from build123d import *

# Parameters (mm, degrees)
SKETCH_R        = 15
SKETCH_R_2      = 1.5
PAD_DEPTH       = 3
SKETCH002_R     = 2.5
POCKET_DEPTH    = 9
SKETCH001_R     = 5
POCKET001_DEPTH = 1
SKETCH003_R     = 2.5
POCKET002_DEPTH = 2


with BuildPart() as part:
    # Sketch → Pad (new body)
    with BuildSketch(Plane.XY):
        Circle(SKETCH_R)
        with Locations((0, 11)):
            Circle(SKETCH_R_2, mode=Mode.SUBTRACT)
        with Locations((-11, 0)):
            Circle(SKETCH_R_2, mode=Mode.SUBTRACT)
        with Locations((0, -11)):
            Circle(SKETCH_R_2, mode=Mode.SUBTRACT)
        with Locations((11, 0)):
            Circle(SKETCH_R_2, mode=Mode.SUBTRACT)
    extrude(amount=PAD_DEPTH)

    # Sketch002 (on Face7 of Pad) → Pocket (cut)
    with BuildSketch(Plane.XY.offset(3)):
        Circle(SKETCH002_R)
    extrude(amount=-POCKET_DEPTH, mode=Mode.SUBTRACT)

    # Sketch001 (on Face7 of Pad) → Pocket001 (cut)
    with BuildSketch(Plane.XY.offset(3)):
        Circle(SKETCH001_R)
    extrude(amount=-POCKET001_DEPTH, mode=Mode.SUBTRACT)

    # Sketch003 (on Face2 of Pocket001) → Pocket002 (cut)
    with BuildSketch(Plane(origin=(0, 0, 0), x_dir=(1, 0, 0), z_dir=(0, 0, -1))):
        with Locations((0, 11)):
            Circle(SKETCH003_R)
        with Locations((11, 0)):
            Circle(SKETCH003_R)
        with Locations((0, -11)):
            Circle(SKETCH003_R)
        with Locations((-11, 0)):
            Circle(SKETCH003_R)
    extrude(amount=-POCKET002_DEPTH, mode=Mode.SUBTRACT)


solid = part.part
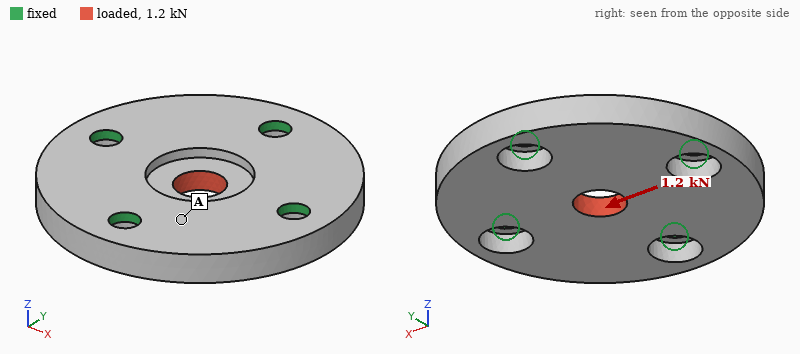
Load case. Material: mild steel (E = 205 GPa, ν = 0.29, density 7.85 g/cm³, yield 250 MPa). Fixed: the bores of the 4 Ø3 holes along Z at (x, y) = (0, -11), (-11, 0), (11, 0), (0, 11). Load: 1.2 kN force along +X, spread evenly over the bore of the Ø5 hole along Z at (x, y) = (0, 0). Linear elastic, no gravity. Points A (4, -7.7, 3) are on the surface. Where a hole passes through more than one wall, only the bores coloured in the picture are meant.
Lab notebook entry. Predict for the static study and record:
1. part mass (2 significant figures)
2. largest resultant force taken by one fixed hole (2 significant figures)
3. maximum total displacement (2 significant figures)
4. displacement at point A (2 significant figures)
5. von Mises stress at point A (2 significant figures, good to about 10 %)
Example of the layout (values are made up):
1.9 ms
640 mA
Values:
14 g
370 N
1.8 µm
0.51 µm
13 MPa
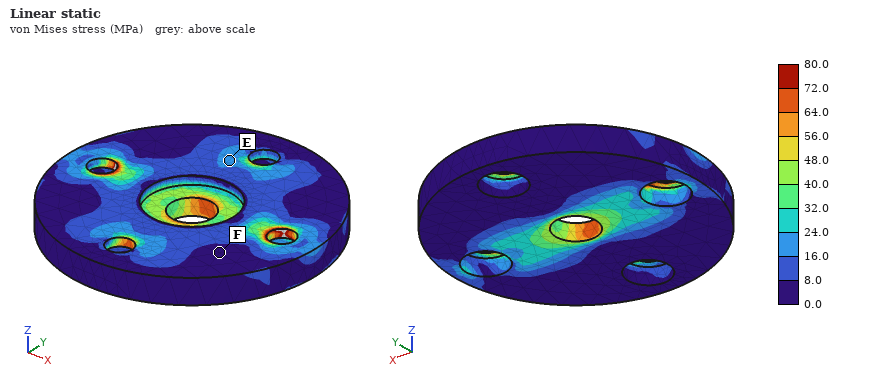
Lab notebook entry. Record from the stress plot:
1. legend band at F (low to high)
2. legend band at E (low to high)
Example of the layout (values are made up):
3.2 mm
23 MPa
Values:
0.0 to 8.0 MPa
16.0 to 24.0 MPa
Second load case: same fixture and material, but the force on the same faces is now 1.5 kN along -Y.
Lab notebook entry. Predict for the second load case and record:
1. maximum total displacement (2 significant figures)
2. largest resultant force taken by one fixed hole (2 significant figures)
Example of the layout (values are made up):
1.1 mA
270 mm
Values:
2.2 µm
470 N
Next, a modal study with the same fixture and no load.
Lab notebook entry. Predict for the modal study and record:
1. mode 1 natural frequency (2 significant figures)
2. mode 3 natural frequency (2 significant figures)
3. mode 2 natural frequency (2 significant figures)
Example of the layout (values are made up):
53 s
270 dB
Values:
26 kHz
29 kHz
29 kHz
